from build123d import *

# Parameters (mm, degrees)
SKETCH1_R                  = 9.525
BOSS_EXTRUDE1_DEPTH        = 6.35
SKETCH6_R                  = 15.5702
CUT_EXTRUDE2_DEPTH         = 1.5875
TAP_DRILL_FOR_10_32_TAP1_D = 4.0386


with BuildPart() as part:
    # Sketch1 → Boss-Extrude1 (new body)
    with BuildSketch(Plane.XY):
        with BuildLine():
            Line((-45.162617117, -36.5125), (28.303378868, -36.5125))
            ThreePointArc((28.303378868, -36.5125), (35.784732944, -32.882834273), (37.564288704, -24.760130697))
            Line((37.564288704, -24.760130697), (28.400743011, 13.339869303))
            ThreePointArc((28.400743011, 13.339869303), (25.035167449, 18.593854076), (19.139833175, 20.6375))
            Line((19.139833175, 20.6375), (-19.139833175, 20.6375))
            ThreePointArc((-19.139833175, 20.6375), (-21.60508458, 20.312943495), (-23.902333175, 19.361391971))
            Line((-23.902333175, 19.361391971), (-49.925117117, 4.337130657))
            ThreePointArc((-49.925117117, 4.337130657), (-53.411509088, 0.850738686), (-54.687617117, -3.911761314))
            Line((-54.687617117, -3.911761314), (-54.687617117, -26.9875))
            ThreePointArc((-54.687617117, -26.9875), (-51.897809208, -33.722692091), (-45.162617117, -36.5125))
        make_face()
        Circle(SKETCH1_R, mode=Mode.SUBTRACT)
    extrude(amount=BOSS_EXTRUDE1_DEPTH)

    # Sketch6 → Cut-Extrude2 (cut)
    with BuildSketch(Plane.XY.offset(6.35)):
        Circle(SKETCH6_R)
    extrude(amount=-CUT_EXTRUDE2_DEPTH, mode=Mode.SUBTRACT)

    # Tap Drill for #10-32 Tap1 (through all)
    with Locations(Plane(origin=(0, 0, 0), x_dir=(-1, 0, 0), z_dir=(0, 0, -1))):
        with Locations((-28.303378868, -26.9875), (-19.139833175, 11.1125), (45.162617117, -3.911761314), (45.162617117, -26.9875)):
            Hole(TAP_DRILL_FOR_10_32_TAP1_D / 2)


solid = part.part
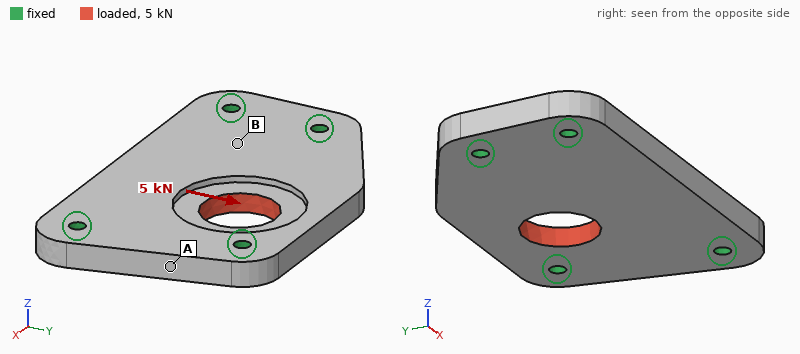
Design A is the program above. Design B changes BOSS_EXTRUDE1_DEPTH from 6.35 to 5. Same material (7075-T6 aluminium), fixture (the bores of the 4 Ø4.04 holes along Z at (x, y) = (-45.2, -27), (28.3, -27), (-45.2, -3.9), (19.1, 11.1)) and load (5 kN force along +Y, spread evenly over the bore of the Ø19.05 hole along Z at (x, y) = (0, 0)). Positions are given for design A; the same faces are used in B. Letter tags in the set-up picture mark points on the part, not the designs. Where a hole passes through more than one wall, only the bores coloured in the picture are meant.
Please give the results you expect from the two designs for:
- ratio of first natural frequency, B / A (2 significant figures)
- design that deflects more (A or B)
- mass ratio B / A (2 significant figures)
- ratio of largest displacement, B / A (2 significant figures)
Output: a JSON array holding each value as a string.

["0.83", "B", "0.81", "1.1"]
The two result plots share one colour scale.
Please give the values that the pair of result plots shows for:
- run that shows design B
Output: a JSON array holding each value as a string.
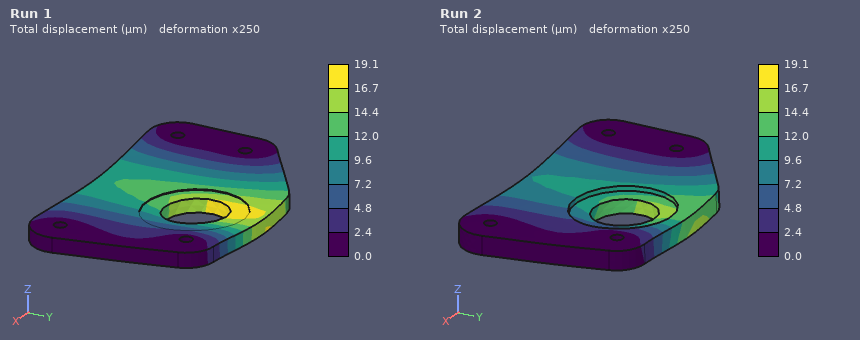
["Run 1"]
